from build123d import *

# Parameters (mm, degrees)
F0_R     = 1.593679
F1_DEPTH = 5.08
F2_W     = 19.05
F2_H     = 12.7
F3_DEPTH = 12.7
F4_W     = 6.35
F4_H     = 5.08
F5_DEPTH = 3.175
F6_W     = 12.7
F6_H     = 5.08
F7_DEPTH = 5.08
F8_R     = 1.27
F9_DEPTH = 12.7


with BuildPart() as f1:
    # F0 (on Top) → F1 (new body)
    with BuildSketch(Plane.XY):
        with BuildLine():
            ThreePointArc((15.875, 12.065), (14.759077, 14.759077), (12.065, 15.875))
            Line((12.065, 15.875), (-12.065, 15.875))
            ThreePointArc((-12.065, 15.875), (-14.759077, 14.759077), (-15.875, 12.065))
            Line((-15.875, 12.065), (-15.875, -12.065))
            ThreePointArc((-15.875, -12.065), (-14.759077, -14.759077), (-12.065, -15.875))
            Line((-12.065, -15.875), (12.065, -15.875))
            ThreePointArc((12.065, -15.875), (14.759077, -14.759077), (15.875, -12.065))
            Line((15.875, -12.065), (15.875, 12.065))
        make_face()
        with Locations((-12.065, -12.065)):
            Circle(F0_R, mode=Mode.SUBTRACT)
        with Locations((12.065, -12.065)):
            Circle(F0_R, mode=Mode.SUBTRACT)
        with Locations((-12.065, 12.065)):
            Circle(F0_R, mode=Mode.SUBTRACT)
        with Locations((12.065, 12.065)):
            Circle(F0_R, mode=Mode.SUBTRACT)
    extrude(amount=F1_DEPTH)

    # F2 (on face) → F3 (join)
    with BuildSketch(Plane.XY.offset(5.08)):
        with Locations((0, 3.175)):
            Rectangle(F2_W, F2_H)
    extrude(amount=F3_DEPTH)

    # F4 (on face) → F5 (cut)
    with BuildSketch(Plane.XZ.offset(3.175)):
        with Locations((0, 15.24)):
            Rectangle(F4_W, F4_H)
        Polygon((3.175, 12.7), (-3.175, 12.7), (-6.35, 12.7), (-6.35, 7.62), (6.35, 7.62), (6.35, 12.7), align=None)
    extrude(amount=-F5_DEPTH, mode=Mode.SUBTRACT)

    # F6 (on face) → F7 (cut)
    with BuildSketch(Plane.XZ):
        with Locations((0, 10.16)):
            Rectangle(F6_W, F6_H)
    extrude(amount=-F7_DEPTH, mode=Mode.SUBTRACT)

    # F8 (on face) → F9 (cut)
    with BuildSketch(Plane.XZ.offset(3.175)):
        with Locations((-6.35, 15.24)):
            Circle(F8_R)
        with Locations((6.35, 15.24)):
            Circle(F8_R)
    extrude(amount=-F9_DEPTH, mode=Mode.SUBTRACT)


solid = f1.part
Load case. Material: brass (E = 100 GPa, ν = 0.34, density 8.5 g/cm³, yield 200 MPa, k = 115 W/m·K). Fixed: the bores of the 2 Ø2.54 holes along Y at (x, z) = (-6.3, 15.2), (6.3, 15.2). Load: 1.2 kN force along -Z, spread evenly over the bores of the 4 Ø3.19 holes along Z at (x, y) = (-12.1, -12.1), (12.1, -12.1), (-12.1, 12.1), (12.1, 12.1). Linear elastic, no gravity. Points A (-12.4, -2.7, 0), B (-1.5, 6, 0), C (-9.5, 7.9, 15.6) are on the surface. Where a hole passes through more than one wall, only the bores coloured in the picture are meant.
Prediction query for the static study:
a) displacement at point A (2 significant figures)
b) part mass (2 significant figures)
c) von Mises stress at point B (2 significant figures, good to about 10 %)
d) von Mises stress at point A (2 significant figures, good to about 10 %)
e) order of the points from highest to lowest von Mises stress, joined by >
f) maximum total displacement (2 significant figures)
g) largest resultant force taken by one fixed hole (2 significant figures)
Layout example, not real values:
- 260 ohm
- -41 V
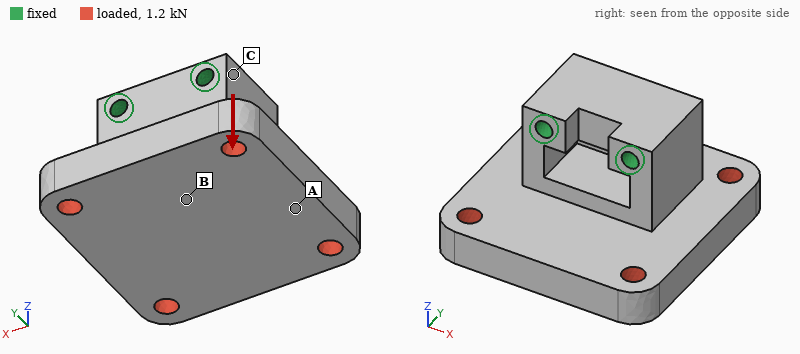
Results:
- 7.4 µm
- 61 g
- 11 MPa
- 33 MPa
- A > B > C
- 26 µm
- 600 N
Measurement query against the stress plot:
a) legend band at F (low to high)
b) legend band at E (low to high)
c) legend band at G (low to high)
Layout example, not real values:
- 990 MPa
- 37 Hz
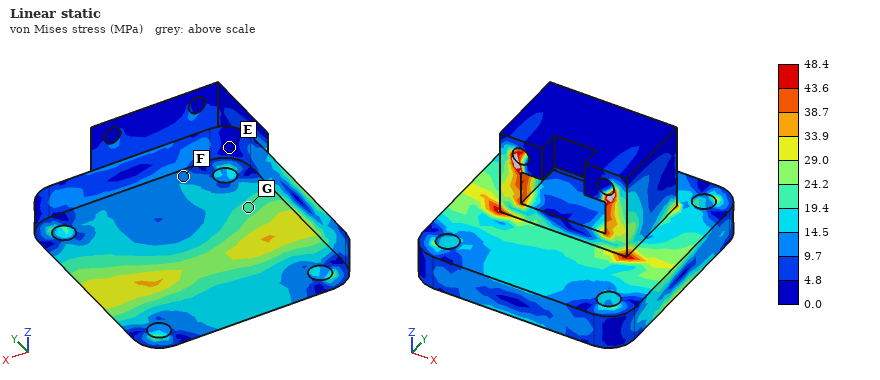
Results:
- 9.7 to 14.5 MPa
- 0.0 to 4.8 MPa
- 19.4 to 24.2 MPa
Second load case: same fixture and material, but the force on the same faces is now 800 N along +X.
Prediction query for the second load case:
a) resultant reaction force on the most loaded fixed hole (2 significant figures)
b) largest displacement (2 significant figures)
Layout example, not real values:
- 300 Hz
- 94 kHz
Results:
- 760 N
- 12 µm
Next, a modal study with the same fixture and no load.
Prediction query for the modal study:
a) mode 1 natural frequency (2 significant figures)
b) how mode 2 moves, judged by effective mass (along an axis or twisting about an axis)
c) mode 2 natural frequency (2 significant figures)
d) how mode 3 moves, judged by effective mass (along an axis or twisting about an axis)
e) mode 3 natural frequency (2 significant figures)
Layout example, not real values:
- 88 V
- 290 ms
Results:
- 6400 Hz
- along X
- 6700 Hz
- along X
- 11 kHz
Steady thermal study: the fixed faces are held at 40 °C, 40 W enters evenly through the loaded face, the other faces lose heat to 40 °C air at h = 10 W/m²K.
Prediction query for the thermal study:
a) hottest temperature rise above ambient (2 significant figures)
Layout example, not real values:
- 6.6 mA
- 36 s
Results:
- 46 K
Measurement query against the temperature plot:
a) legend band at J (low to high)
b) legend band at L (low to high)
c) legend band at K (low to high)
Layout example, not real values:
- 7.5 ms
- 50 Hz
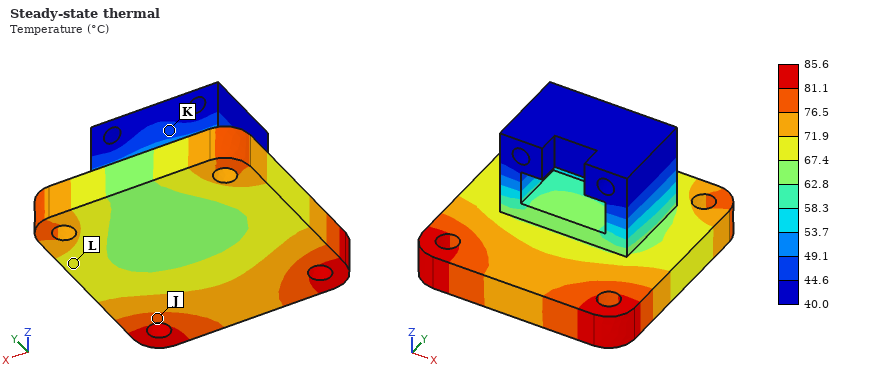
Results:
- 76.5 to 81.1 °C
- 67.4 to 71.9 °C
- 44.6 to 49.1 °C
